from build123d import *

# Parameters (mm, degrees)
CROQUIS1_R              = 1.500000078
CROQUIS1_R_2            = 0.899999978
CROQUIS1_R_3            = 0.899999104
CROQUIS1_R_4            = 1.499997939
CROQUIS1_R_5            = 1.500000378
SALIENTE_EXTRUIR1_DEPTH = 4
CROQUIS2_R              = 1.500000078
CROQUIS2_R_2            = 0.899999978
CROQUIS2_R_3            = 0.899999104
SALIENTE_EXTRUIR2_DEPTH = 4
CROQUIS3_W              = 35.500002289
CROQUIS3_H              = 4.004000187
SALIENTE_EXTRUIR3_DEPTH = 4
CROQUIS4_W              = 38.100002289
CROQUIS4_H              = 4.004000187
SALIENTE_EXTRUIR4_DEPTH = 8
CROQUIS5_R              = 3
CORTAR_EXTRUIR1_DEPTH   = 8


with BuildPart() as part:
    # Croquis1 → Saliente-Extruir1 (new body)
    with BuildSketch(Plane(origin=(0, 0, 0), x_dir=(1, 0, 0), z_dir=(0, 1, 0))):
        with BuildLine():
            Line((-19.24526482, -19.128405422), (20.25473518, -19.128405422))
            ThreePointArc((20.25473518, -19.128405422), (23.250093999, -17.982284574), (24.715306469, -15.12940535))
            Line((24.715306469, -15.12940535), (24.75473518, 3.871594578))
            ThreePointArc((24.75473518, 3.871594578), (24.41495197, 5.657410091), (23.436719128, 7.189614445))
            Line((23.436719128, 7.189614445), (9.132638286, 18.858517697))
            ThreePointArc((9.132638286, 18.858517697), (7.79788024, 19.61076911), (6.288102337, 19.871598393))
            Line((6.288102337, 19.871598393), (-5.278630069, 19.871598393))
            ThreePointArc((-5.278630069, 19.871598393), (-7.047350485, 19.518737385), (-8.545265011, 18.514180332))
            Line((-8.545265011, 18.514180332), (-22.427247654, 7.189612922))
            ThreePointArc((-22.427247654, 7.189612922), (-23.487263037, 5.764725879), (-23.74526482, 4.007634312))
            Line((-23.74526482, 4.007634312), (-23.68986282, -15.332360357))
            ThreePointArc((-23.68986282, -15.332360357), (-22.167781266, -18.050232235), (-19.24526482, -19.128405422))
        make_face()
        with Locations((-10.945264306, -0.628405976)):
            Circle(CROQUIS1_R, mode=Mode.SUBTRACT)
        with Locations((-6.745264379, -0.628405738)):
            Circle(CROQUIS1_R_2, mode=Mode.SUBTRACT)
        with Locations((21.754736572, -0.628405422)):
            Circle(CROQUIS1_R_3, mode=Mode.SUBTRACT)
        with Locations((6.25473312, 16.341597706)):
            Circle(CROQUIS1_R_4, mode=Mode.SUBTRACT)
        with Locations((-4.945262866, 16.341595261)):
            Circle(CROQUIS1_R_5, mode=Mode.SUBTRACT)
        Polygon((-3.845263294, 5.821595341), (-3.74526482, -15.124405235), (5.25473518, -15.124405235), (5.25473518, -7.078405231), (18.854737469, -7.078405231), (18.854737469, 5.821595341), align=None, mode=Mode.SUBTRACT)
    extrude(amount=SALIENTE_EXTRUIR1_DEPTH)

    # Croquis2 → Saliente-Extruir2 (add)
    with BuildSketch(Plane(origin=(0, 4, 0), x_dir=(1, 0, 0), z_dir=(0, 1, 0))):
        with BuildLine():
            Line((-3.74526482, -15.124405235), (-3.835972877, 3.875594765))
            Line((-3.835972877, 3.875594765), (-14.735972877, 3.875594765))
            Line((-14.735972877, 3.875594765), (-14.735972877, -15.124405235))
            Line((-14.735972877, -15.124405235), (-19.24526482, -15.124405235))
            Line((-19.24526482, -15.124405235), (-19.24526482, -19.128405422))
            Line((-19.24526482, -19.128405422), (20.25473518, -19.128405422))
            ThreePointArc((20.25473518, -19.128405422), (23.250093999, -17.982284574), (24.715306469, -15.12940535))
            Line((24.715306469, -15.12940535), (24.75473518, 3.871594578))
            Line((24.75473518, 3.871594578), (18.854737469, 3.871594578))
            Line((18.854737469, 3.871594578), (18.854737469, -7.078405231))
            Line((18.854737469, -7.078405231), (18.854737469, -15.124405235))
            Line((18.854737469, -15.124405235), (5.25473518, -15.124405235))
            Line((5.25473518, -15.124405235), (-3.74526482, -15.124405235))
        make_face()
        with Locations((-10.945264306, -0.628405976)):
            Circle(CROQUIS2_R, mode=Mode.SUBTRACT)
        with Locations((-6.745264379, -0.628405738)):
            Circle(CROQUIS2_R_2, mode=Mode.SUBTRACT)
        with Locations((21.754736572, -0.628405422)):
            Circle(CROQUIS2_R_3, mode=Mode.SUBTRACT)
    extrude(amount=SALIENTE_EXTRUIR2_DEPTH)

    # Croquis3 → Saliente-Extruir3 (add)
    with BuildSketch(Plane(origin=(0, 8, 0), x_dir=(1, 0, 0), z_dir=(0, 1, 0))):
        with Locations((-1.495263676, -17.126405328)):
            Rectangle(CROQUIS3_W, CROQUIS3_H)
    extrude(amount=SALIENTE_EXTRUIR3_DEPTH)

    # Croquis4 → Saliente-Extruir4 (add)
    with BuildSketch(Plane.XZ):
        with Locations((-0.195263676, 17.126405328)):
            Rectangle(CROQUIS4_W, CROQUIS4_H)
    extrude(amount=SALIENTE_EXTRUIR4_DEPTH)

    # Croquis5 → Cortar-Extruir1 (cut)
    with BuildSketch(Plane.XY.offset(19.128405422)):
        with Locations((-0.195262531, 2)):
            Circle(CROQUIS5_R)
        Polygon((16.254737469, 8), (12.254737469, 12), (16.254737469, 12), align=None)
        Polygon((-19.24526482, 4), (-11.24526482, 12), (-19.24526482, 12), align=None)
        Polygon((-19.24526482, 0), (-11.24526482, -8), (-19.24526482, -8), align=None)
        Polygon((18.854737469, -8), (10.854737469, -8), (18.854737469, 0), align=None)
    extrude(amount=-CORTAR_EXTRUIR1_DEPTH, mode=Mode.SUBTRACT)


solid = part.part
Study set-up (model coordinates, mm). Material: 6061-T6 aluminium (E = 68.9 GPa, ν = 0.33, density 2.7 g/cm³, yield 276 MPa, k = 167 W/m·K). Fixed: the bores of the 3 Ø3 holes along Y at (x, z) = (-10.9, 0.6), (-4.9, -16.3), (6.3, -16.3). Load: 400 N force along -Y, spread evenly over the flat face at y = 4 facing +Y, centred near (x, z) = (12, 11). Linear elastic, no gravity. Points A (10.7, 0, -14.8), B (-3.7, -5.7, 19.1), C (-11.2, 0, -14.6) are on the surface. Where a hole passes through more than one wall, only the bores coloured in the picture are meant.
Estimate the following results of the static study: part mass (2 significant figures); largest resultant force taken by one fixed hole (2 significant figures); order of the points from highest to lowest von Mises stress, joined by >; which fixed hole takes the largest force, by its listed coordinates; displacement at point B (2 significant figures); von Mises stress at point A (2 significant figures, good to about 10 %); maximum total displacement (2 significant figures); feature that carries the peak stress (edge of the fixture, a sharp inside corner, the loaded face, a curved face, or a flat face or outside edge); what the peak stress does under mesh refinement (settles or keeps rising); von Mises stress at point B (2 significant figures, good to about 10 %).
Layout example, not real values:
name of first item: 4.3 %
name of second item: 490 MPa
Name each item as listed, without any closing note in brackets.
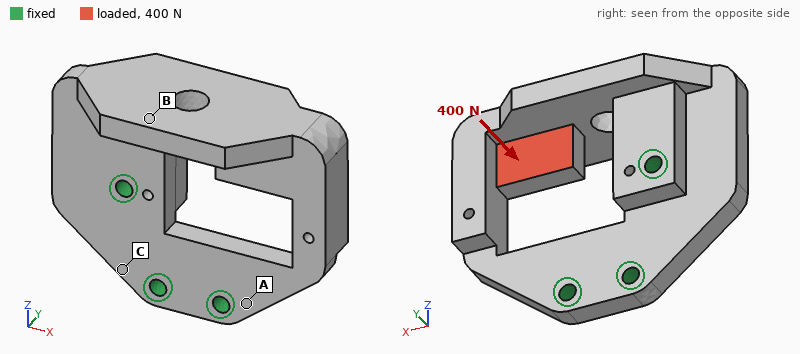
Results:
part mass: 22 g
largest resultant force taken by one fixed hole: 310 N
order of the points from highest to lowest von Mises stress, joined by >: A > B > C
which fixed hole takes the largest force, by its listed coordinates: (-10.9, 0.6)
displacement at point B: 0.047 mm
von Mises stress at point A: 46 MPa
maximum total displacement: 0.12 mm
feature that carries the peak stress: edge of the fixture
what the peak stress does under mesh refinement: keeps rising
von Mises stress at point B: 19 MPa
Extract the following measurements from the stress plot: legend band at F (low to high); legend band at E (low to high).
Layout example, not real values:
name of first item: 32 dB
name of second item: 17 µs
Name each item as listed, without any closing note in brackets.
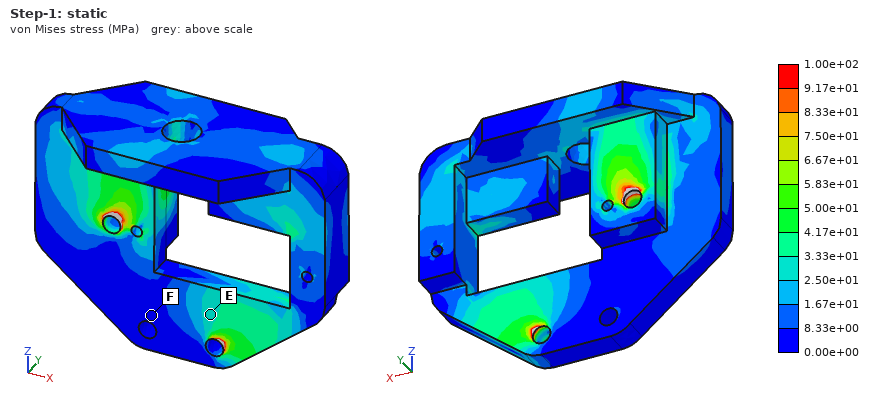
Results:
legend band at F: 0.00e+00 to 8.33e+00 MPa
legend band at E: 2.50e+01 to 3.33e+01 MPa
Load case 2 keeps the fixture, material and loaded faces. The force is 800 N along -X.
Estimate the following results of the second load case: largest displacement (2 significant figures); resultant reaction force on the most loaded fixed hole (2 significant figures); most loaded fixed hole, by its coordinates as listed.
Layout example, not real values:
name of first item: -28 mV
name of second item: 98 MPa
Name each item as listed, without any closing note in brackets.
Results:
largest displacement: 34 µm
resultant reaction force on the most loaded fixed hole: 1.1 kN
most loaded fixed hole, by its coordinates as listed: (-10.9, 0.6)
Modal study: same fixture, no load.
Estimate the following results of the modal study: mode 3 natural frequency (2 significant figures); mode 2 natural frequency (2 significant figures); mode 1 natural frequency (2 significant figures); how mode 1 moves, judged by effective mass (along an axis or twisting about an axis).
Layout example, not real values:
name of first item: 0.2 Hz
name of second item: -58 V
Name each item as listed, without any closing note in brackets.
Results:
mode 3 natural frequency: 8500 Hz
mode 2 natural frequency: 7700 Hz
mode 1 natural frequency: 3600 Hz
how mode 1 moves, judged by effective mass: along Y
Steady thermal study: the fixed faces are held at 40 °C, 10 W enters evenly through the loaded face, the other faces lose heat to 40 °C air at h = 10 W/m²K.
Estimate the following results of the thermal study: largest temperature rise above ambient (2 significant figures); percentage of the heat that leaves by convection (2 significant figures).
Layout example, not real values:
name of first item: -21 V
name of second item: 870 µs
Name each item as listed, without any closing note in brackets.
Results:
largest temperature rise above ambient: 22 K
percentage of the heat that leaves by convection: 3.7 %
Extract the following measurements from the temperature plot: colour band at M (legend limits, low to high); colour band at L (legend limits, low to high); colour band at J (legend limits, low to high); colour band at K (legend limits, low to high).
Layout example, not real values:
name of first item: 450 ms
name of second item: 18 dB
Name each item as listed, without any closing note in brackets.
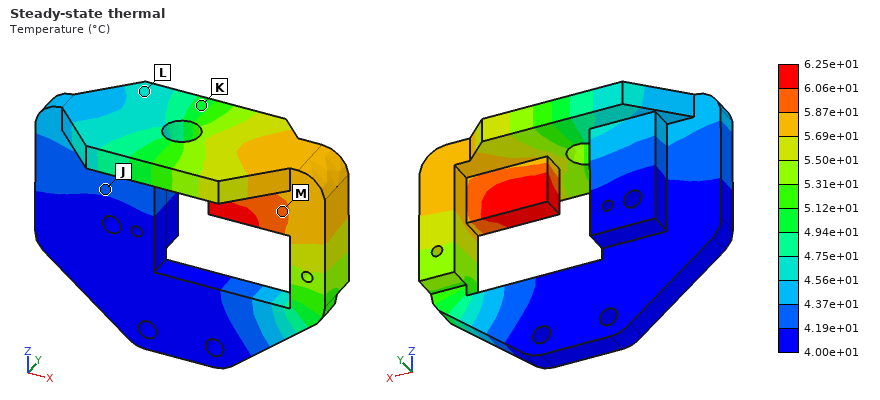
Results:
colour band at M: 5.87e+01 to 6.06e+01 °C
colour band at L: 4.56e+01 to 4.75e+01 °C
colour band at J: 4.19e+01 to 4.37e+01 °C
colour band at K: 4.94e+01 to 5.12e+01 °C
